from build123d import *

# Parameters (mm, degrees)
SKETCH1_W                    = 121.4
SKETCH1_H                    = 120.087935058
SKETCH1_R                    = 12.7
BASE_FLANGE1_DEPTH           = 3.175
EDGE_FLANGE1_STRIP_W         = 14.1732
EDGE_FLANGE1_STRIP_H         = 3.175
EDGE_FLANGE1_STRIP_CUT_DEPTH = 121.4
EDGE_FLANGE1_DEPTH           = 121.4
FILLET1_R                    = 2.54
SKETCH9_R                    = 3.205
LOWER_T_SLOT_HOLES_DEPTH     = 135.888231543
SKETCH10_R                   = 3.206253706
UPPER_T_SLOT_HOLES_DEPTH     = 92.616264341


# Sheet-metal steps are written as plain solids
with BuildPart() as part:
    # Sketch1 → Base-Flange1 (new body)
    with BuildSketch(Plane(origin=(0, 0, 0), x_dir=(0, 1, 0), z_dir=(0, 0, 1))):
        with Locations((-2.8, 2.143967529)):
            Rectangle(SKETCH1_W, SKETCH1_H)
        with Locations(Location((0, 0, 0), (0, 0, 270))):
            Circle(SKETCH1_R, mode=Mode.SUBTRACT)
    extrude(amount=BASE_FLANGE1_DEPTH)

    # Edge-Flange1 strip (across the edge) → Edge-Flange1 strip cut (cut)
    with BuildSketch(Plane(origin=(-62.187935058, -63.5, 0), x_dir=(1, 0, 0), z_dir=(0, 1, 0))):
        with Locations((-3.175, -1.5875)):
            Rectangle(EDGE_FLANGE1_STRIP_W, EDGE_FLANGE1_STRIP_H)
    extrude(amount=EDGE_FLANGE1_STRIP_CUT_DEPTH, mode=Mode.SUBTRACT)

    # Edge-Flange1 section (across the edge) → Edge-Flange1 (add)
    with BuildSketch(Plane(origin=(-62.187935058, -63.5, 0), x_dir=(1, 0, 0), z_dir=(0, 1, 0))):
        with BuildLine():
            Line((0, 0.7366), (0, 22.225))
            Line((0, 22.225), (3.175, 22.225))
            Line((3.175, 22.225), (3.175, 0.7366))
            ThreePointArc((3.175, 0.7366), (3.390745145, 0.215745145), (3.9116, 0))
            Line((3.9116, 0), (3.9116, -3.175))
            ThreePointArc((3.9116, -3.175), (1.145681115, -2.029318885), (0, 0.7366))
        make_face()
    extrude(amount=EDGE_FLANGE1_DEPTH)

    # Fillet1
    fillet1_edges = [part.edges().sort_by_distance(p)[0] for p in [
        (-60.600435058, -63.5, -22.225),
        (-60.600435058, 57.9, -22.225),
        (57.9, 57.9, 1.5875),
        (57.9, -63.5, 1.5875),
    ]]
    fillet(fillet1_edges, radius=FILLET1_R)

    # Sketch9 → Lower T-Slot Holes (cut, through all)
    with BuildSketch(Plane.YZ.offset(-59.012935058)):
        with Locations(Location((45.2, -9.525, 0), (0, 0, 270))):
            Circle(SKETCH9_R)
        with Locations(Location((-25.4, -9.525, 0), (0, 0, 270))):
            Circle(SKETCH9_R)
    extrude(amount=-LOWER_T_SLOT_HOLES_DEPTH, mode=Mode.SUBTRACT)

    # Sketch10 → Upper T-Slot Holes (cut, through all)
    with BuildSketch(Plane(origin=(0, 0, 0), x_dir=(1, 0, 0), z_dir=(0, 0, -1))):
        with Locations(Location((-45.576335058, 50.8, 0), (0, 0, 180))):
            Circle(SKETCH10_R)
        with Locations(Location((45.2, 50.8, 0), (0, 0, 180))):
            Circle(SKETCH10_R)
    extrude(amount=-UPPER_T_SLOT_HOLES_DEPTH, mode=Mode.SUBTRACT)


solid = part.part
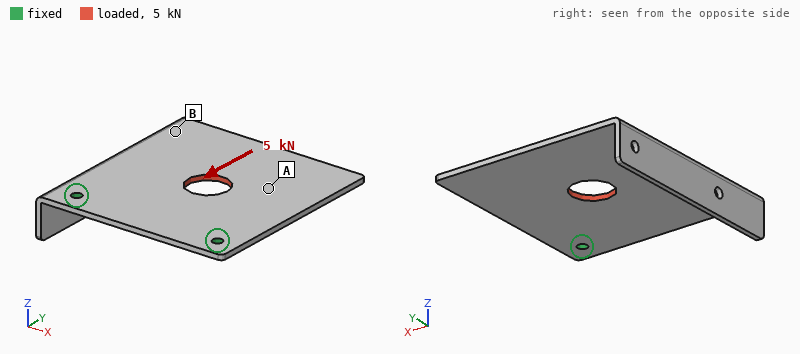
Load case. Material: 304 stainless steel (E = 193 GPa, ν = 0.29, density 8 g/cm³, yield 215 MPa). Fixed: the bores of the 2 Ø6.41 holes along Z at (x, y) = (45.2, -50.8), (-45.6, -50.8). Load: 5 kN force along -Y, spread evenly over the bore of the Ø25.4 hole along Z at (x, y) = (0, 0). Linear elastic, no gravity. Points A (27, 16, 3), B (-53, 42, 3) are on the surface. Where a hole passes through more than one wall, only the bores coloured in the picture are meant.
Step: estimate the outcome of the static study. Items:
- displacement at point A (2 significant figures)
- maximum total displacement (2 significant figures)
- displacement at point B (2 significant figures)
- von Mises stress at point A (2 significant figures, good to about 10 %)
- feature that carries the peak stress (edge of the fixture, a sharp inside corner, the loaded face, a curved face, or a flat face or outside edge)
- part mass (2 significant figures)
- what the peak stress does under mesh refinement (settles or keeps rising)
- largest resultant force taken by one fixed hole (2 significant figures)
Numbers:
7.7 µm
11 µm
9.1 µm
12 MPa
edge of the fixture
420 g
keeps rising
2.6 kN
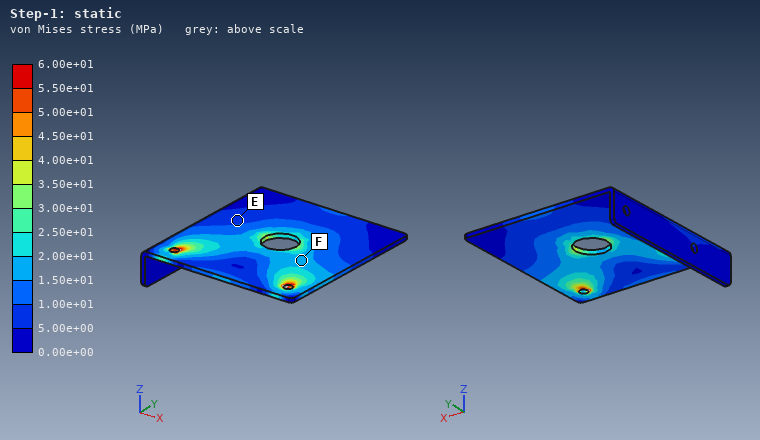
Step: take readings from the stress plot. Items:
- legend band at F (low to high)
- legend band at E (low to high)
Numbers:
1.50e+01 to 2.00e+01 MPa
5.00e+00 to 1.00e+01 MPa
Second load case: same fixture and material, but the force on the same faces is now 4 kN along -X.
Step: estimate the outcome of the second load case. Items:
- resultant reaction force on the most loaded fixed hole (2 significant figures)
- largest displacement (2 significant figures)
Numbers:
2.9 kN
22 µm
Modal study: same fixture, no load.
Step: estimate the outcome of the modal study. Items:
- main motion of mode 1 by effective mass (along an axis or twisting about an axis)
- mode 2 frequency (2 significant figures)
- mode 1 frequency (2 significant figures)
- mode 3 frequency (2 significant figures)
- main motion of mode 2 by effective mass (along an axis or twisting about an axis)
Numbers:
along Z
460 Hz
250 Hz
1100 Hz
twisting about Y
